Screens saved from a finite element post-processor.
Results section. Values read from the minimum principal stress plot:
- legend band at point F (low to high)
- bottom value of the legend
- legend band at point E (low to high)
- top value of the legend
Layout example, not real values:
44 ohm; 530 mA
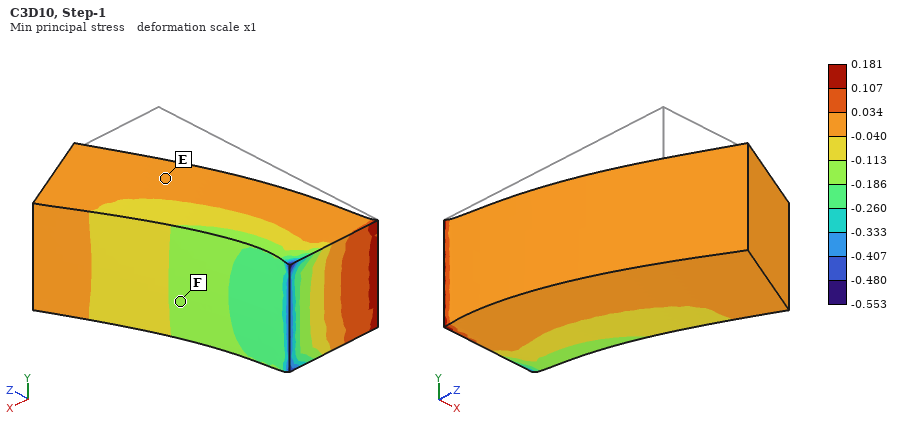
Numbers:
-0.186 to -0.113; -0.553; -0.040 to 0.034; 0.181
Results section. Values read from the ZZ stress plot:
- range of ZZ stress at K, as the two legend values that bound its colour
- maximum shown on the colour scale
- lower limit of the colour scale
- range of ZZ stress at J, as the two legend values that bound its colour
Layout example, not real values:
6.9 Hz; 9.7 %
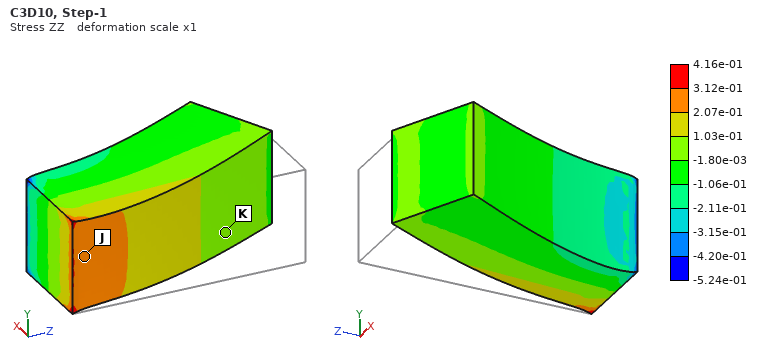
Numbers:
-1.80e-03 to 1.03e-01; 4.16e-01; -5.24e-01; 2.07e-01 to 3.12e-01
